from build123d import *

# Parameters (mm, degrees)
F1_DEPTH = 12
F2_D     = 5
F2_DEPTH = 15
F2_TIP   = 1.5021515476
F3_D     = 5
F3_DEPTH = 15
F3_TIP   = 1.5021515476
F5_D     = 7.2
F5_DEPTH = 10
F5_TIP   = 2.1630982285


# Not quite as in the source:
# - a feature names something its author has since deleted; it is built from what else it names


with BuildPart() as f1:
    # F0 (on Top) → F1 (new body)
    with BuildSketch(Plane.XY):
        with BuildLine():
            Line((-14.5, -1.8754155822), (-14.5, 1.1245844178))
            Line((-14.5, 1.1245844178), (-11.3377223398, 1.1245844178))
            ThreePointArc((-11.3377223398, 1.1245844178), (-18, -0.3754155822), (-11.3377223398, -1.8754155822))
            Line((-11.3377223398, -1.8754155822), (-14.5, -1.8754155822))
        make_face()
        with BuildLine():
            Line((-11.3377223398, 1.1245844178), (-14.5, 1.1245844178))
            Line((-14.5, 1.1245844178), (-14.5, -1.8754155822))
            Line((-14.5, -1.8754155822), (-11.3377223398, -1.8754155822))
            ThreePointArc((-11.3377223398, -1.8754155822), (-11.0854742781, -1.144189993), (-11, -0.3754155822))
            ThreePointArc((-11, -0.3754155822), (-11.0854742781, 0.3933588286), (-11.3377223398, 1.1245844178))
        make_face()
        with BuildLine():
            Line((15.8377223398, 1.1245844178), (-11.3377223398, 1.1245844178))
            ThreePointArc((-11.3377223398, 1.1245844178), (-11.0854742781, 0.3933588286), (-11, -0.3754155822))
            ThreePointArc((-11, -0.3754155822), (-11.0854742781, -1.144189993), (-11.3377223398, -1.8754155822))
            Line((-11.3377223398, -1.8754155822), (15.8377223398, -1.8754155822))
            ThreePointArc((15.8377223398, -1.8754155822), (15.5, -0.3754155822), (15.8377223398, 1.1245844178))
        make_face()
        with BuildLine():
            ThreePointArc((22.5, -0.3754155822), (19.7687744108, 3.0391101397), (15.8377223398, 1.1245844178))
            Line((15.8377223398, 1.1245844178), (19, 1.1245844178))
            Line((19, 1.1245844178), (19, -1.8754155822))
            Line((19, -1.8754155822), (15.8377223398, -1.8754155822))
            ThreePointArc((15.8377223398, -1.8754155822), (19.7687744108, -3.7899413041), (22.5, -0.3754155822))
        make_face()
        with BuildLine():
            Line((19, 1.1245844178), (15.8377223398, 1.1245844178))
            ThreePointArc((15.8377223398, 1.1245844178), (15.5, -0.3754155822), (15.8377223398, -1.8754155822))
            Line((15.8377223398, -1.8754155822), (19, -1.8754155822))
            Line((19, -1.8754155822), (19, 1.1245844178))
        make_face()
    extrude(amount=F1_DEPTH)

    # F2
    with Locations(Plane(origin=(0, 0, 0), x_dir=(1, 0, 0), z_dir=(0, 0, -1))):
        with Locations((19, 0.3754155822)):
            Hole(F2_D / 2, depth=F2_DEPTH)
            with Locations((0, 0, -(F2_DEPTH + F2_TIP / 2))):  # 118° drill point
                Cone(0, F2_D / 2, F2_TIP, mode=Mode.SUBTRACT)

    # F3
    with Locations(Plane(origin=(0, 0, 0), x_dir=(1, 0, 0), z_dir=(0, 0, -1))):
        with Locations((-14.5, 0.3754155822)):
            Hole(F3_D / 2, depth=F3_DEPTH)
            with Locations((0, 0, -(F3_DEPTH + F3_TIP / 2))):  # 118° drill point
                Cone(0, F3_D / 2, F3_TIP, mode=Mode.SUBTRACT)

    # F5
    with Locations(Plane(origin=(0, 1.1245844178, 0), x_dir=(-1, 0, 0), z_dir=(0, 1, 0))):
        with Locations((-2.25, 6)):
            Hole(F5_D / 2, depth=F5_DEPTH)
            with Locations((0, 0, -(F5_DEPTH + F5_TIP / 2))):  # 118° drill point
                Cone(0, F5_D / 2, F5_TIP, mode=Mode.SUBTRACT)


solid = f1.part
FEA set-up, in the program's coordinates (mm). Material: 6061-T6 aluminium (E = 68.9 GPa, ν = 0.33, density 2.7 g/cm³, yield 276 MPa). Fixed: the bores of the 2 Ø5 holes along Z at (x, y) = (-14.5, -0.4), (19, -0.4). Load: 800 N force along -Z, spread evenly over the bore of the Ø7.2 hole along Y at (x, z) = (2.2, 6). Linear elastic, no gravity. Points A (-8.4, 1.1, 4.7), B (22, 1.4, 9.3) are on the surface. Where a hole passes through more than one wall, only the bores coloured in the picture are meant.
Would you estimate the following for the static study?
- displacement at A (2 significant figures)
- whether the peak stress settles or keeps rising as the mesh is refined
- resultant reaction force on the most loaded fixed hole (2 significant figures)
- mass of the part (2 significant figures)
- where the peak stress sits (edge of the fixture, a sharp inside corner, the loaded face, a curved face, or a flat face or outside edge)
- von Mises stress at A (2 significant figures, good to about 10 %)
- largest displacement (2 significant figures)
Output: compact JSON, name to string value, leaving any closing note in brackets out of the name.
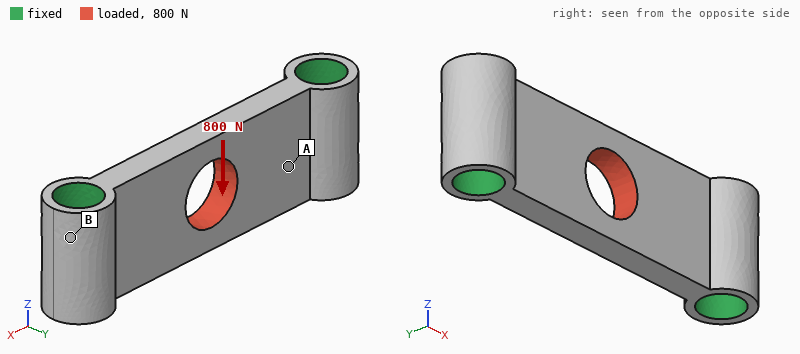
{"displacement at A": "2.2 µm", "whether the peak stress settles or keeps rising as the mesh is refined": "keeps rising", "resultant reaction force on the most loaded fixed hole": "400 N", "mass of the part": "3.5 g", "where the peak stress sits": "edge of the fixture", "von Mises stress at A": "27 MPa", "largest displacement": "10 µm"}
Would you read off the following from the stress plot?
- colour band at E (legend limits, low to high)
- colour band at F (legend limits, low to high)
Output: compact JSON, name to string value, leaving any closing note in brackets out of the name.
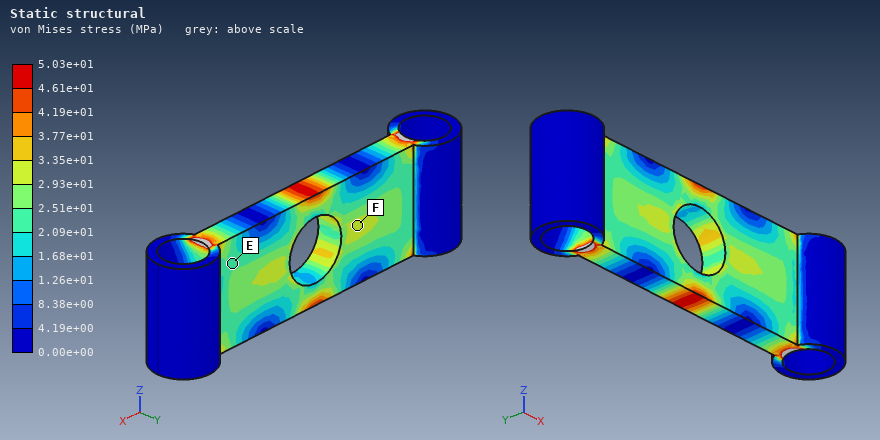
{"colour band at E": "2.09e+01 to 2.51e+01 MPa", "colour band at F": "2.93e+01 to 3.35e+01 MPa"}
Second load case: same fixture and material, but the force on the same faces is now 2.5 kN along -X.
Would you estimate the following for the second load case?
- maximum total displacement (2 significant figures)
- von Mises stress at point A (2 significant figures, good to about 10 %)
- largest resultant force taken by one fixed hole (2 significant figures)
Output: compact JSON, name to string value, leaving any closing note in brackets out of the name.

{"maximum total displacement": "7.3 µm", "von Mises stress at point A": "34 MPa", "largest resultant force taken by one fixed hole": "1.3 kN"}
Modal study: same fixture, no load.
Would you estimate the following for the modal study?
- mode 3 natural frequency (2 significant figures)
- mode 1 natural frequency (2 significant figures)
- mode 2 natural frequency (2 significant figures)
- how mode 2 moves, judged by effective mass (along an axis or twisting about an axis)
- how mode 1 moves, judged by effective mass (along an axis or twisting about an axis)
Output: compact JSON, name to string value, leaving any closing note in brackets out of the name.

{"mode 3 natural frequency": "44 kHz", "mode 1 natural frequency": "19 kHz", "mode 2 natural frequency": "30 kHz", "how mode 2 moves, judged by effective mass": "twisting about X", "how mode 1 moves, judged by effective mass": "along Y"}
